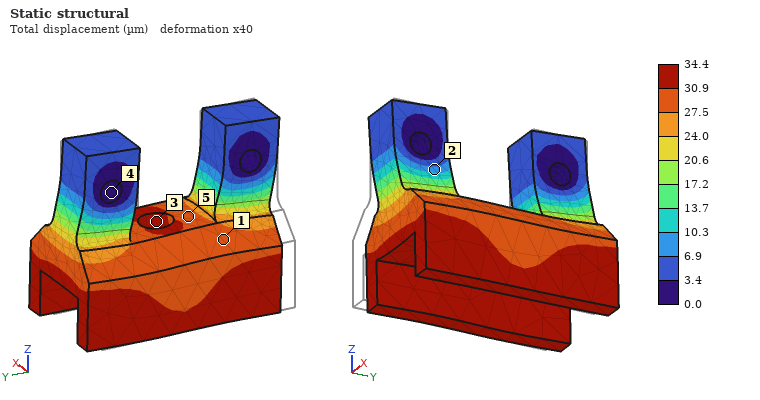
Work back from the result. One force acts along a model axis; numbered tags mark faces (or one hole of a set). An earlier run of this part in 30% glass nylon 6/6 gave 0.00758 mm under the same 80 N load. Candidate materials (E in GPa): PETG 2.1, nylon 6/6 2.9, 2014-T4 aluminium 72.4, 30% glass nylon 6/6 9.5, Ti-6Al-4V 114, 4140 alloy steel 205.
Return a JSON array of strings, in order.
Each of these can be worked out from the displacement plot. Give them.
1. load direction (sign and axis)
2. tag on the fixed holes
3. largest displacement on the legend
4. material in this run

["+Y", "4", "34.4 µm", "PETG"]
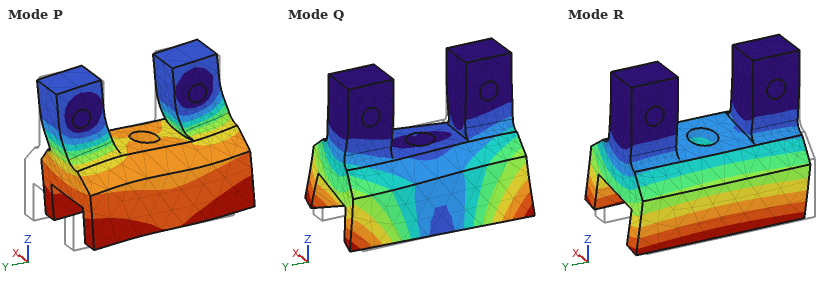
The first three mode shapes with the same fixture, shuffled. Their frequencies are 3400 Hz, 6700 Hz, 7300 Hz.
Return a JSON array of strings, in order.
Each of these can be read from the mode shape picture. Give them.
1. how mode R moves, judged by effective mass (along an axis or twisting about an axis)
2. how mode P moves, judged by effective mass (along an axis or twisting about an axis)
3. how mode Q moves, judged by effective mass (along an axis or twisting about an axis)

["along X", "along Y", "twisting about Z"]
